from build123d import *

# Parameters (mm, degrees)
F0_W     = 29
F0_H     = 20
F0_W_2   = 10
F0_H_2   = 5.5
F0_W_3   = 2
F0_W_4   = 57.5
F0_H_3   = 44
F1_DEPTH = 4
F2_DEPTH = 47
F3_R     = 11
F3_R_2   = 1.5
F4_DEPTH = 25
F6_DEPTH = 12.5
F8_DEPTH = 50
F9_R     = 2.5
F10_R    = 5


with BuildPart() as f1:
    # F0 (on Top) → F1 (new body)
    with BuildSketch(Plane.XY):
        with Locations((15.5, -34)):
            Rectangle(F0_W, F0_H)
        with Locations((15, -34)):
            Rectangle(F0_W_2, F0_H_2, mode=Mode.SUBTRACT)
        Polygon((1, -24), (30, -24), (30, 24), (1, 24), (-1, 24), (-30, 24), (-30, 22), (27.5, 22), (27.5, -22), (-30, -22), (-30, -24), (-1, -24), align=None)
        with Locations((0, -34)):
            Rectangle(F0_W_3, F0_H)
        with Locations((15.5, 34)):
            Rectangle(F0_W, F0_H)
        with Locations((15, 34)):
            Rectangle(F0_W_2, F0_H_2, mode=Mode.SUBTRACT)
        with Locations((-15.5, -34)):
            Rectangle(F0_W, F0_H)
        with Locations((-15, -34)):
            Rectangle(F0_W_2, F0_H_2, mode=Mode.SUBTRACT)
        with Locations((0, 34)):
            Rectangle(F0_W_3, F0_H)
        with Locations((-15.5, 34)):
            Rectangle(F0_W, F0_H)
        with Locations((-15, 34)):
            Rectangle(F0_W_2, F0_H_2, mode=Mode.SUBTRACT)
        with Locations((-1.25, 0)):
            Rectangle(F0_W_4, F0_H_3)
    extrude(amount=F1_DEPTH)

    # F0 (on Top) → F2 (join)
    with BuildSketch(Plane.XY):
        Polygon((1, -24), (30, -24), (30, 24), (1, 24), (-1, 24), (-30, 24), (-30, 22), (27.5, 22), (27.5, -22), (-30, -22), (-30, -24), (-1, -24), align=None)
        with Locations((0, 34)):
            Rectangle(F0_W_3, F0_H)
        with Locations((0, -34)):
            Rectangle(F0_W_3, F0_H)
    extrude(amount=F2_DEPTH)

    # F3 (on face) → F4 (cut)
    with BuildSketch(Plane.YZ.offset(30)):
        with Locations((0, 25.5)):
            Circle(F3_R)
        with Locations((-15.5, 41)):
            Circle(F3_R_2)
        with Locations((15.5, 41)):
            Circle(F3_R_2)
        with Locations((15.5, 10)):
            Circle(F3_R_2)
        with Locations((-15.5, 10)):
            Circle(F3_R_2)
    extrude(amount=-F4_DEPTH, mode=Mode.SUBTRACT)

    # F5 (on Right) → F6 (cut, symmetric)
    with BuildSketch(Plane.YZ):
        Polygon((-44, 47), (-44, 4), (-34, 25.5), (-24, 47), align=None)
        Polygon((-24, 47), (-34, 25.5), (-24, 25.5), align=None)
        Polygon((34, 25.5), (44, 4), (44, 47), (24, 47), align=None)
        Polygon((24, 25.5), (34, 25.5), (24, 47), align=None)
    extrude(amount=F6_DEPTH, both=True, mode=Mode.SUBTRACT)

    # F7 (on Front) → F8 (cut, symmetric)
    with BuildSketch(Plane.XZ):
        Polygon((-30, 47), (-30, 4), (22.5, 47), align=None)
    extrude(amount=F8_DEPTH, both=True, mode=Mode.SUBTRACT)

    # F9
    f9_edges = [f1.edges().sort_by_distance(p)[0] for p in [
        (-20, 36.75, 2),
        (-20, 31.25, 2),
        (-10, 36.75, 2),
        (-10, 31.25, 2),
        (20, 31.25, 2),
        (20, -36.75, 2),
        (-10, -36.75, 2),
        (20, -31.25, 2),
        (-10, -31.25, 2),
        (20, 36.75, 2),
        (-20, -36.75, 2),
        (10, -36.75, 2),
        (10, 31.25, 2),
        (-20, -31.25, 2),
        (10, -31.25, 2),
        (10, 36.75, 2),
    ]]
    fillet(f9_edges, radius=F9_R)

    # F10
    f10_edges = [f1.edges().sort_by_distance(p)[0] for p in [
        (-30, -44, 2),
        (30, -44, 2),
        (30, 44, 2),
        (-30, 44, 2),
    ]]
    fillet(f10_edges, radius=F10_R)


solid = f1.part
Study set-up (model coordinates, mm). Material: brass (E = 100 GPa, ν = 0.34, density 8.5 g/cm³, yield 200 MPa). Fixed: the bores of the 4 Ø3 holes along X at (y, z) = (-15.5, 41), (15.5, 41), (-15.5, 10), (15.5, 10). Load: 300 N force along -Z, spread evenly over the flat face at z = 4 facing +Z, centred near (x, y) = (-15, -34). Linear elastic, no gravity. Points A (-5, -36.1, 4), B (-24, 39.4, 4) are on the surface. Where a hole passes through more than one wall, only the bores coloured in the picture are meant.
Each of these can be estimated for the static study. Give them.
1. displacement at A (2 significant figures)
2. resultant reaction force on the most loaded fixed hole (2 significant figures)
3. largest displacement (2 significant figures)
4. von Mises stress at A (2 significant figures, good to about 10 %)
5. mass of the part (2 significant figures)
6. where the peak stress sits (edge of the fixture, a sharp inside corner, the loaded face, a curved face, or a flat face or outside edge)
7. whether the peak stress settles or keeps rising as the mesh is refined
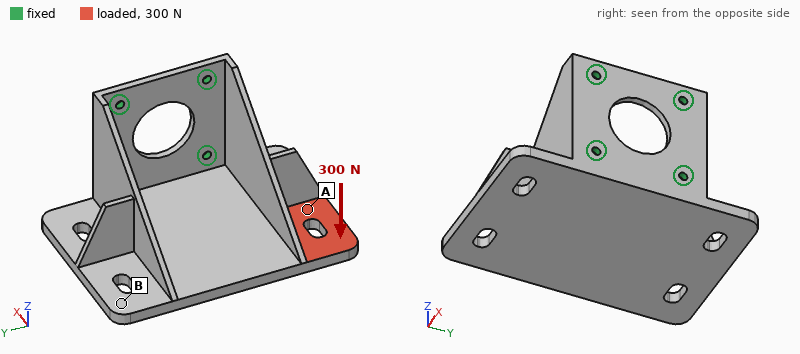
0.067 mm
480 N
0.13 mm
18 MPa
260 g
edge of the fixture
keeps rising
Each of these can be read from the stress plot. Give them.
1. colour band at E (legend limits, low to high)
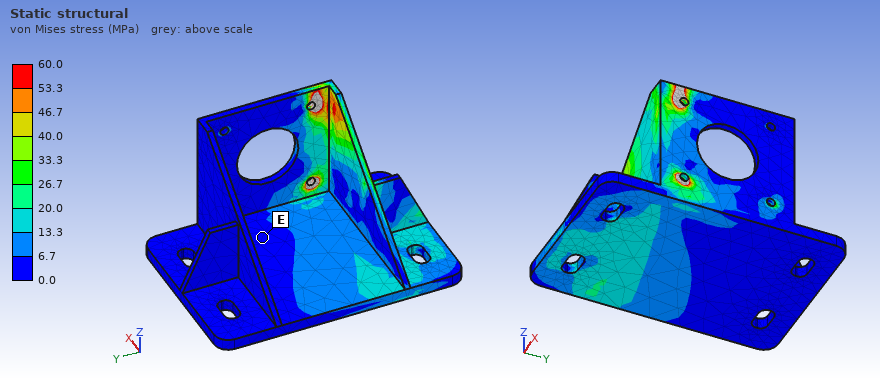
0.0 to 6.7 MPa
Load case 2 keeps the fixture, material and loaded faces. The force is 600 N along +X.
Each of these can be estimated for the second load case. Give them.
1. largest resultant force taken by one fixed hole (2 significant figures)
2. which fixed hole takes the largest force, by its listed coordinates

940 N
(-15.5, 10)
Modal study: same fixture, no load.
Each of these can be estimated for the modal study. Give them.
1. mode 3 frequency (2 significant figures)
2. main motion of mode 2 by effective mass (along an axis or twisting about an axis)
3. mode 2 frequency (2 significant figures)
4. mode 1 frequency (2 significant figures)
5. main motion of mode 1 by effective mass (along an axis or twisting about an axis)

2200 Hz
along Z
1500 Hz
1100 Hz
along Y
